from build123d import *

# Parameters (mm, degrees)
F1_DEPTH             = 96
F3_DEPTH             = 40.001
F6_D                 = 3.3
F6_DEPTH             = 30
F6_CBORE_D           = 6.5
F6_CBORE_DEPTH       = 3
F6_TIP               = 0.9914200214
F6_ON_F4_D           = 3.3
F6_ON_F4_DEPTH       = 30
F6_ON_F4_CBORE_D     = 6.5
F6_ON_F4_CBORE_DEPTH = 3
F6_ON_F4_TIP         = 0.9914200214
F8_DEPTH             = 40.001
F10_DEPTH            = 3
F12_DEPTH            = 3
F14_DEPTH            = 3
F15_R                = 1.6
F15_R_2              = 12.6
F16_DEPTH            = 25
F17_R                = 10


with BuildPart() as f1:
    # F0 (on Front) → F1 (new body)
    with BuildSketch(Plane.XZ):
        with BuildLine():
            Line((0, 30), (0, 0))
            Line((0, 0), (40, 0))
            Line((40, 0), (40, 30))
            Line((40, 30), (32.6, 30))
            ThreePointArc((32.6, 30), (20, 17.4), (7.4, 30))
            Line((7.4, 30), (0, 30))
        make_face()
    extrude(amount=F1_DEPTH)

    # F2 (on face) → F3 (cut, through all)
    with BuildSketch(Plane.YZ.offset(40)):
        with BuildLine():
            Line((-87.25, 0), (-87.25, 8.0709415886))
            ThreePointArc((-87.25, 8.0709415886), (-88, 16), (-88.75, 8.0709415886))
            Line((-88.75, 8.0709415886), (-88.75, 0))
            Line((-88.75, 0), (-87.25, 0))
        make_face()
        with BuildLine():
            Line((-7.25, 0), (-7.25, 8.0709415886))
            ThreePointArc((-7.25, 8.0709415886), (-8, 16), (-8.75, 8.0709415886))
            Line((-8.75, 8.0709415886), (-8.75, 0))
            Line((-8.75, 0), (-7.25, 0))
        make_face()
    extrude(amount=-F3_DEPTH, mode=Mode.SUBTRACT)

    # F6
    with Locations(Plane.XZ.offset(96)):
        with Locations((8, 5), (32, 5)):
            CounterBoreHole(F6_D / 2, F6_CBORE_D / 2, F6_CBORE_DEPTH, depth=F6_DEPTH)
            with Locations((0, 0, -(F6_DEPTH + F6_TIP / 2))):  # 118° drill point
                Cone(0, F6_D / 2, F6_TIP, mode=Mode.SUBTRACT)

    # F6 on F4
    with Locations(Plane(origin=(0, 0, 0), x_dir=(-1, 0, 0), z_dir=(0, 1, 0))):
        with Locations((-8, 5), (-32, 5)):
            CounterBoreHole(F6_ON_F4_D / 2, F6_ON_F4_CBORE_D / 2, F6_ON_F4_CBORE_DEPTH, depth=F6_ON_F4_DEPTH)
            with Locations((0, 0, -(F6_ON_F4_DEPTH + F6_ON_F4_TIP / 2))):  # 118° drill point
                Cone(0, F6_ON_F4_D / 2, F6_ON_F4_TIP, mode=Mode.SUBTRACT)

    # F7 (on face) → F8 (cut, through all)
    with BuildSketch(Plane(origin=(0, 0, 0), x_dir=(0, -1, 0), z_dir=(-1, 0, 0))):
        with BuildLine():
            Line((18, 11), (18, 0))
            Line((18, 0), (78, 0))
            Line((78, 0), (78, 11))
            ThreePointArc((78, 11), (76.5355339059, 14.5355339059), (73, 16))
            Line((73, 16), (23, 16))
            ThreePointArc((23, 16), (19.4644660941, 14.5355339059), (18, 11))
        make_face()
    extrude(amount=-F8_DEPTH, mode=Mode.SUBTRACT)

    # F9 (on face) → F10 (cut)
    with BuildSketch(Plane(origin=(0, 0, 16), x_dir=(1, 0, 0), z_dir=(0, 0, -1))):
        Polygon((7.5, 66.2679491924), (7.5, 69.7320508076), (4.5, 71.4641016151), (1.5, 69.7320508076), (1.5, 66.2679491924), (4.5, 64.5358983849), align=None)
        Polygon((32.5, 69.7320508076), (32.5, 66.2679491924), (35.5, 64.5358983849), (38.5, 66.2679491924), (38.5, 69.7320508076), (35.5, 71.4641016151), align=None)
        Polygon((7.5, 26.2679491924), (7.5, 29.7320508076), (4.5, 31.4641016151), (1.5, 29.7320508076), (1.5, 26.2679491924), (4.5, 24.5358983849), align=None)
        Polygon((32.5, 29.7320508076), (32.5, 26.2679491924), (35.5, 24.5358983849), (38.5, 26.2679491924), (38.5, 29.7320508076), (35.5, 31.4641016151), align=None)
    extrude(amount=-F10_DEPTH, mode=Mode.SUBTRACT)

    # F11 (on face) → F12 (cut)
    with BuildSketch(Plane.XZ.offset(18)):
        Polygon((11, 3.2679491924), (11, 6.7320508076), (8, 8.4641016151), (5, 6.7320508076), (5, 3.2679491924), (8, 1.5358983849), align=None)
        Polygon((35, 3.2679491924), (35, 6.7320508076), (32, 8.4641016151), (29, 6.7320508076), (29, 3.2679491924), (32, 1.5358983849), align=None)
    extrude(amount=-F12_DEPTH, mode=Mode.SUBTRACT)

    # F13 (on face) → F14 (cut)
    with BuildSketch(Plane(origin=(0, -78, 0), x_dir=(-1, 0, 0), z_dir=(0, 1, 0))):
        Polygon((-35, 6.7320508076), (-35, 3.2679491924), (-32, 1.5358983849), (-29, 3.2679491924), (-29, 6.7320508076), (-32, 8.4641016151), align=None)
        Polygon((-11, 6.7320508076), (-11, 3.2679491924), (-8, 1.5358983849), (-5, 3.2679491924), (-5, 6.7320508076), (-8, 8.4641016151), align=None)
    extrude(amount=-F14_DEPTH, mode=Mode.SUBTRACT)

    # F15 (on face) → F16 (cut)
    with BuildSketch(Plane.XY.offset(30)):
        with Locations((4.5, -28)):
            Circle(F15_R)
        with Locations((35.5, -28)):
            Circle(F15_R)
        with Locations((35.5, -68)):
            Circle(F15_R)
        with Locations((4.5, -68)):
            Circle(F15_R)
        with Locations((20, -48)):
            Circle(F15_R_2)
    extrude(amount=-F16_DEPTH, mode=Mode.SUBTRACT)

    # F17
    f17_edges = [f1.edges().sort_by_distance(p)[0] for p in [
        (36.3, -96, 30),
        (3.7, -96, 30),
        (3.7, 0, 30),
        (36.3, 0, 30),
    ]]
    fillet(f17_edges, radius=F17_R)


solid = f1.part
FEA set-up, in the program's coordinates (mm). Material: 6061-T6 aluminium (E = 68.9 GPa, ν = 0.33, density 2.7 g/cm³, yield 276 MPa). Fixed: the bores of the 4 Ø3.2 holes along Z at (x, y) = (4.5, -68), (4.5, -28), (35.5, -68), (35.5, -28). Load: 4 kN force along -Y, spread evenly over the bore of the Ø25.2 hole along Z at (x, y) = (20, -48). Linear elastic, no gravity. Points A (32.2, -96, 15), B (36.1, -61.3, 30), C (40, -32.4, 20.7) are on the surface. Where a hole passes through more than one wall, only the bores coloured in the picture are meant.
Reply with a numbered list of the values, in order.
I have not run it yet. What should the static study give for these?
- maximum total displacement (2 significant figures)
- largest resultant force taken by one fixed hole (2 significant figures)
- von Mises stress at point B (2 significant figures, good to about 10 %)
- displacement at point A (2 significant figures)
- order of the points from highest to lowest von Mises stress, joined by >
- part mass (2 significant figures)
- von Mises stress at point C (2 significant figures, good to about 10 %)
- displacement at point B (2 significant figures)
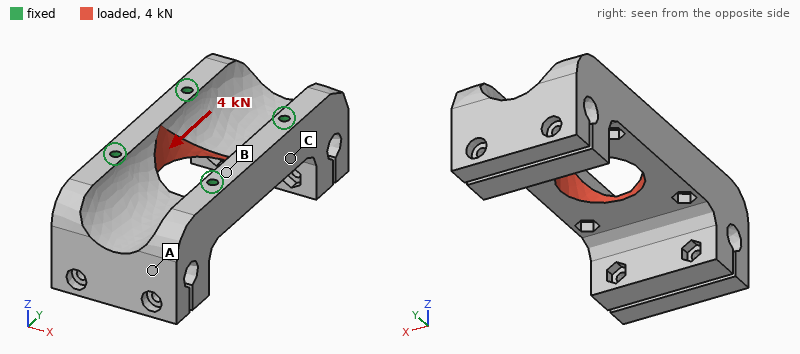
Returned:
1. 3.7 µm
2. 1.0 kN
3. 6.6 MPa
4. 2.7 µm
5. B > C > A
6. 120 g
7. 4.3 MPa
8. 0.68 µm
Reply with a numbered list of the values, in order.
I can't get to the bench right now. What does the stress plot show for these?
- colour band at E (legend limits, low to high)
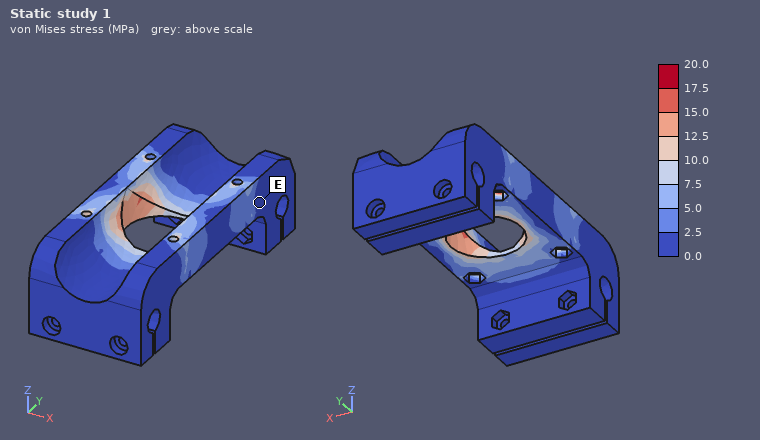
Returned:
1. 0.0 to 2.5 MPa
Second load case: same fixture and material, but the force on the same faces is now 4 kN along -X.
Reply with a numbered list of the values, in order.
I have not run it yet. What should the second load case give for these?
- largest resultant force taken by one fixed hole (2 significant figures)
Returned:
1. 1.0 kN
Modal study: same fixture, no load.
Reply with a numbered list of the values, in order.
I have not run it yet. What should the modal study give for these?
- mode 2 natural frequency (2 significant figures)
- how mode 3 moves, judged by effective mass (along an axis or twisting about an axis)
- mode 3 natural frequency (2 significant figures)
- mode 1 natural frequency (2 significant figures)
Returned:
1. 5300 Hz
2. twisting about Y
3. 8400 Hz
4. 5200 Hz
